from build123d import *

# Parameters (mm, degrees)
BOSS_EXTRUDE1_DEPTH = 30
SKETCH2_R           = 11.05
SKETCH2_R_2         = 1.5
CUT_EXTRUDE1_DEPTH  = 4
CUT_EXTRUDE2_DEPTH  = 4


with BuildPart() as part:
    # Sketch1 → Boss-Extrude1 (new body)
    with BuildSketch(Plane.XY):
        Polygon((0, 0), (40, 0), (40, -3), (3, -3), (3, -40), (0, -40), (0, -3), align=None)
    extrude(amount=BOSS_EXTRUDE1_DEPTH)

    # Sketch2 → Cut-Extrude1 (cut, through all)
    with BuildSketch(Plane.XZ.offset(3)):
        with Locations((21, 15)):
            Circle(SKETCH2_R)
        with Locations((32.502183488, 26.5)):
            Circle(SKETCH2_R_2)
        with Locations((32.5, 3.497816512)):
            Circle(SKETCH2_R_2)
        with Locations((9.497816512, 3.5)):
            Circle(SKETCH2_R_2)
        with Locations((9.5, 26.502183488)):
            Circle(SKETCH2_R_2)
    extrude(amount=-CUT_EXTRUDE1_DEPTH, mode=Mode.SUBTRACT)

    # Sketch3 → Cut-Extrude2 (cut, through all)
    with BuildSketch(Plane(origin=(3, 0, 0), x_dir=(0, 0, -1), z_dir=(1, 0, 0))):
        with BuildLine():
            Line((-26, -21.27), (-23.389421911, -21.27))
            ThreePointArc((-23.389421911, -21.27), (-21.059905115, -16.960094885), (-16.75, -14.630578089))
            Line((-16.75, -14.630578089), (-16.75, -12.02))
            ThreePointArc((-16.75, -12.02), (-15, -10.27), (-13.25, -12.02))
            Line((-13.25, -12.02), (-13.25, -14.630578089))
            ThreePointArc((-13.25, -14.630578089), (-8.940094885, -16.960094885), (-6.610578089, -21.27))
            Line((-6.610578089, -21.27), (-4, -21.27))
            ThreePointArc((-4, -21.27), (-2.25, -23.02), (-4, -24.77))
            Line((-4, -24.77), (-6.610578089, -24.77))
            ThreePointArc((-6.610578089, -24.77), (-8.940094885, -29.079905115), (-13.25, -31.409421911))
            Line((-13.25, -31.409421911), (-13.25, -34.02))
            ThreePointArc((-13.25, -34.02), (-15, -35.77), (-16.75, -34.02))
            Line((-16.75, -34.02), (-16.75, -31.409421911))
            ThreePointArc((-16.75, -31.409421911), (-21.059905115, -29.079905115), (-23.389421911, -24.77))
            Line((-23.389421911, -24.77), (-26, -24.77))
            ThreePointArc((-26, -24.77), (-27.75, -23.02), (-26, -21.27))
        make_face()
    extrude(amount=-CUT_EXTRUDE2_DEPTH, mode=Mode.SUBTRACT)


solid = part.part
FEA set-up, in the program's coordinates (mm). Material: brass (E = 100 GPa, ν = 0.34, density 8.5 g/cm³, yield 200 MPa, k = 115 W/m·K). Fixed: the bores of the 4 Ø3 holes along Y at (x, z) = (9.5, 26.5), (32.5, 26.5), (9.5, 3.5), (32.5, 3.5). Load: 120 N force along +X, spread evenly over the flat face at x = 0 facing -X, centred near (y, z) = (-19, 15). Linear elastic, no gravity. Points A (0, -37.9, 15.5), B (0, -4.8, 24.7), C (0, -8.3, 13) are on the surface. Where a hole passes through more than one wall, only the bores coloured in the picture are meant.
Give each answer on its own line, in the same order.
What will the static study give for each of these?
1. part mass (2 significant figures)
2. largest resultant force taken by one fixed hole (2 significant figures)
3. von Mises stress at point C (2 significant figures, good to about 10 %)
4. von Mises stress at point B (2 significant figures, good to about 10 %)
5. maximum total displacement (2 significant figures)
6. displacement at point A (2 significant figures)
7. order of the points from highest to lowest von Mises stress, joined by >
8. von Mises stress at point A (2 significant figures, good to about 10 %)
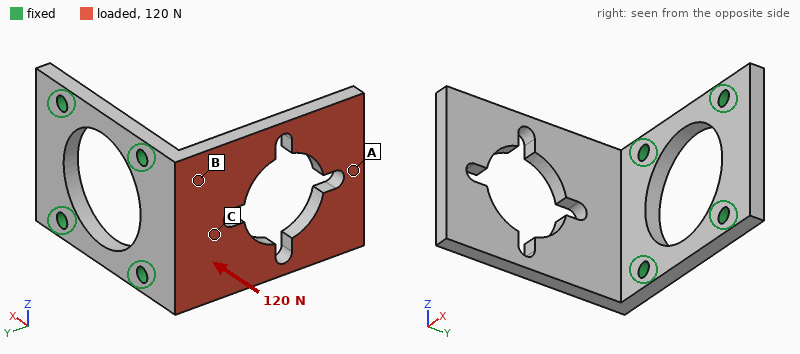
41 g
68 N
24 MPa
37 MPa
0.28 mm
0.26 mm
B > C > A
10 MPa
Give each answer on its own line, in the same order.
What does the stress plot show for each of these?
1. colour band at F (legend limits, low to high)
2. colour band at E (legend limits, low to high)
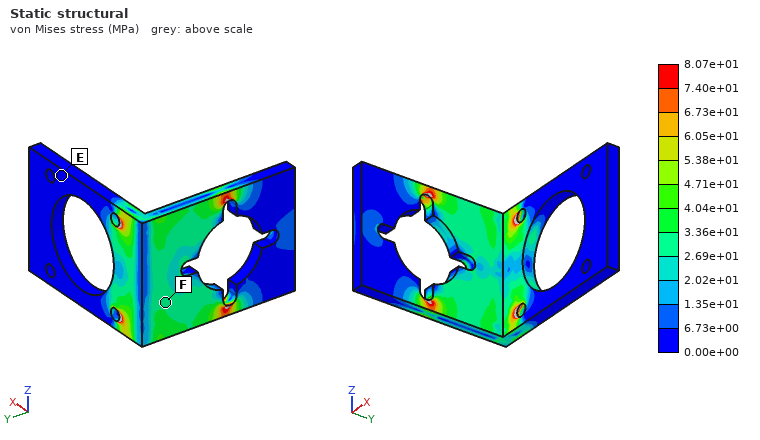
2.69e+01 to 3.36e+01 MPa
0.00e+00 to 6.73e+00 MPa
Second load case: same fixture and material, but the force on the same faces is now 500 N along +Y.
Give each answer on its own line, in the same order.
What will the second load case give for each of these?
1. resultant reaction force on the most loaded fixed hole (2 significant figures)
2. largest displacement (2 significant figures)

250 N
0.23 mm
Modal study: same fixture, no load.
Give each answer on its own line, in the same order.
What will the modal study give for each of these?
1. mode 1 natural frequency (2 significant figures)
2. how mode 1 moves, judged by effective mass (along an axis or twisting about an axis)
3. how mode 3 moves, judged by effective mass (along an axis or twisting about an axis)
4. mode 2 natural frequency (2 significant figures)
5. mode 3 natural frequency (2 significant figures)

820 Hz
along X
along Z
2300 Hz
3300 Hz
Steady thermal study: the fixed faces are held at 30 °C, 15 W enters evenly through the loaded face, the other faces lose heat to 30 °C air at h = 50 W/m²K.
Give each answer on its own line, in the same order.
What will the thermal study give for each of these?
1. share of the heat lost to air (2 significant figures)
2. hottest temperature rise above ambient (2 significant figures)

18 %
51 K
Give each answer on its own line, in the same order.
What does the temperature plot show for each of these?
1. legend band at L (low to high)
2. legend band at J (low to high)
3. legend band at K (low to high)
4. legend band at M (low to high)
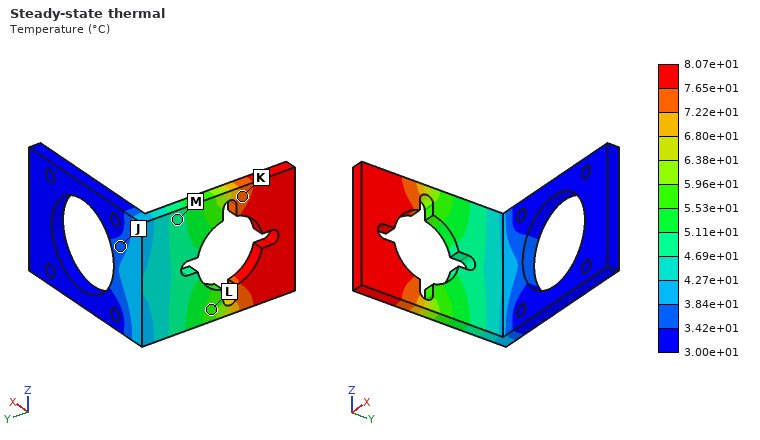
5.53e+01 to 5.96e+01 °C
3.42e+01 to 3.84e+01 °C
7.22e+01 to 7.65e+01 °C
4.69e+01 to 5.11e+01 °C
